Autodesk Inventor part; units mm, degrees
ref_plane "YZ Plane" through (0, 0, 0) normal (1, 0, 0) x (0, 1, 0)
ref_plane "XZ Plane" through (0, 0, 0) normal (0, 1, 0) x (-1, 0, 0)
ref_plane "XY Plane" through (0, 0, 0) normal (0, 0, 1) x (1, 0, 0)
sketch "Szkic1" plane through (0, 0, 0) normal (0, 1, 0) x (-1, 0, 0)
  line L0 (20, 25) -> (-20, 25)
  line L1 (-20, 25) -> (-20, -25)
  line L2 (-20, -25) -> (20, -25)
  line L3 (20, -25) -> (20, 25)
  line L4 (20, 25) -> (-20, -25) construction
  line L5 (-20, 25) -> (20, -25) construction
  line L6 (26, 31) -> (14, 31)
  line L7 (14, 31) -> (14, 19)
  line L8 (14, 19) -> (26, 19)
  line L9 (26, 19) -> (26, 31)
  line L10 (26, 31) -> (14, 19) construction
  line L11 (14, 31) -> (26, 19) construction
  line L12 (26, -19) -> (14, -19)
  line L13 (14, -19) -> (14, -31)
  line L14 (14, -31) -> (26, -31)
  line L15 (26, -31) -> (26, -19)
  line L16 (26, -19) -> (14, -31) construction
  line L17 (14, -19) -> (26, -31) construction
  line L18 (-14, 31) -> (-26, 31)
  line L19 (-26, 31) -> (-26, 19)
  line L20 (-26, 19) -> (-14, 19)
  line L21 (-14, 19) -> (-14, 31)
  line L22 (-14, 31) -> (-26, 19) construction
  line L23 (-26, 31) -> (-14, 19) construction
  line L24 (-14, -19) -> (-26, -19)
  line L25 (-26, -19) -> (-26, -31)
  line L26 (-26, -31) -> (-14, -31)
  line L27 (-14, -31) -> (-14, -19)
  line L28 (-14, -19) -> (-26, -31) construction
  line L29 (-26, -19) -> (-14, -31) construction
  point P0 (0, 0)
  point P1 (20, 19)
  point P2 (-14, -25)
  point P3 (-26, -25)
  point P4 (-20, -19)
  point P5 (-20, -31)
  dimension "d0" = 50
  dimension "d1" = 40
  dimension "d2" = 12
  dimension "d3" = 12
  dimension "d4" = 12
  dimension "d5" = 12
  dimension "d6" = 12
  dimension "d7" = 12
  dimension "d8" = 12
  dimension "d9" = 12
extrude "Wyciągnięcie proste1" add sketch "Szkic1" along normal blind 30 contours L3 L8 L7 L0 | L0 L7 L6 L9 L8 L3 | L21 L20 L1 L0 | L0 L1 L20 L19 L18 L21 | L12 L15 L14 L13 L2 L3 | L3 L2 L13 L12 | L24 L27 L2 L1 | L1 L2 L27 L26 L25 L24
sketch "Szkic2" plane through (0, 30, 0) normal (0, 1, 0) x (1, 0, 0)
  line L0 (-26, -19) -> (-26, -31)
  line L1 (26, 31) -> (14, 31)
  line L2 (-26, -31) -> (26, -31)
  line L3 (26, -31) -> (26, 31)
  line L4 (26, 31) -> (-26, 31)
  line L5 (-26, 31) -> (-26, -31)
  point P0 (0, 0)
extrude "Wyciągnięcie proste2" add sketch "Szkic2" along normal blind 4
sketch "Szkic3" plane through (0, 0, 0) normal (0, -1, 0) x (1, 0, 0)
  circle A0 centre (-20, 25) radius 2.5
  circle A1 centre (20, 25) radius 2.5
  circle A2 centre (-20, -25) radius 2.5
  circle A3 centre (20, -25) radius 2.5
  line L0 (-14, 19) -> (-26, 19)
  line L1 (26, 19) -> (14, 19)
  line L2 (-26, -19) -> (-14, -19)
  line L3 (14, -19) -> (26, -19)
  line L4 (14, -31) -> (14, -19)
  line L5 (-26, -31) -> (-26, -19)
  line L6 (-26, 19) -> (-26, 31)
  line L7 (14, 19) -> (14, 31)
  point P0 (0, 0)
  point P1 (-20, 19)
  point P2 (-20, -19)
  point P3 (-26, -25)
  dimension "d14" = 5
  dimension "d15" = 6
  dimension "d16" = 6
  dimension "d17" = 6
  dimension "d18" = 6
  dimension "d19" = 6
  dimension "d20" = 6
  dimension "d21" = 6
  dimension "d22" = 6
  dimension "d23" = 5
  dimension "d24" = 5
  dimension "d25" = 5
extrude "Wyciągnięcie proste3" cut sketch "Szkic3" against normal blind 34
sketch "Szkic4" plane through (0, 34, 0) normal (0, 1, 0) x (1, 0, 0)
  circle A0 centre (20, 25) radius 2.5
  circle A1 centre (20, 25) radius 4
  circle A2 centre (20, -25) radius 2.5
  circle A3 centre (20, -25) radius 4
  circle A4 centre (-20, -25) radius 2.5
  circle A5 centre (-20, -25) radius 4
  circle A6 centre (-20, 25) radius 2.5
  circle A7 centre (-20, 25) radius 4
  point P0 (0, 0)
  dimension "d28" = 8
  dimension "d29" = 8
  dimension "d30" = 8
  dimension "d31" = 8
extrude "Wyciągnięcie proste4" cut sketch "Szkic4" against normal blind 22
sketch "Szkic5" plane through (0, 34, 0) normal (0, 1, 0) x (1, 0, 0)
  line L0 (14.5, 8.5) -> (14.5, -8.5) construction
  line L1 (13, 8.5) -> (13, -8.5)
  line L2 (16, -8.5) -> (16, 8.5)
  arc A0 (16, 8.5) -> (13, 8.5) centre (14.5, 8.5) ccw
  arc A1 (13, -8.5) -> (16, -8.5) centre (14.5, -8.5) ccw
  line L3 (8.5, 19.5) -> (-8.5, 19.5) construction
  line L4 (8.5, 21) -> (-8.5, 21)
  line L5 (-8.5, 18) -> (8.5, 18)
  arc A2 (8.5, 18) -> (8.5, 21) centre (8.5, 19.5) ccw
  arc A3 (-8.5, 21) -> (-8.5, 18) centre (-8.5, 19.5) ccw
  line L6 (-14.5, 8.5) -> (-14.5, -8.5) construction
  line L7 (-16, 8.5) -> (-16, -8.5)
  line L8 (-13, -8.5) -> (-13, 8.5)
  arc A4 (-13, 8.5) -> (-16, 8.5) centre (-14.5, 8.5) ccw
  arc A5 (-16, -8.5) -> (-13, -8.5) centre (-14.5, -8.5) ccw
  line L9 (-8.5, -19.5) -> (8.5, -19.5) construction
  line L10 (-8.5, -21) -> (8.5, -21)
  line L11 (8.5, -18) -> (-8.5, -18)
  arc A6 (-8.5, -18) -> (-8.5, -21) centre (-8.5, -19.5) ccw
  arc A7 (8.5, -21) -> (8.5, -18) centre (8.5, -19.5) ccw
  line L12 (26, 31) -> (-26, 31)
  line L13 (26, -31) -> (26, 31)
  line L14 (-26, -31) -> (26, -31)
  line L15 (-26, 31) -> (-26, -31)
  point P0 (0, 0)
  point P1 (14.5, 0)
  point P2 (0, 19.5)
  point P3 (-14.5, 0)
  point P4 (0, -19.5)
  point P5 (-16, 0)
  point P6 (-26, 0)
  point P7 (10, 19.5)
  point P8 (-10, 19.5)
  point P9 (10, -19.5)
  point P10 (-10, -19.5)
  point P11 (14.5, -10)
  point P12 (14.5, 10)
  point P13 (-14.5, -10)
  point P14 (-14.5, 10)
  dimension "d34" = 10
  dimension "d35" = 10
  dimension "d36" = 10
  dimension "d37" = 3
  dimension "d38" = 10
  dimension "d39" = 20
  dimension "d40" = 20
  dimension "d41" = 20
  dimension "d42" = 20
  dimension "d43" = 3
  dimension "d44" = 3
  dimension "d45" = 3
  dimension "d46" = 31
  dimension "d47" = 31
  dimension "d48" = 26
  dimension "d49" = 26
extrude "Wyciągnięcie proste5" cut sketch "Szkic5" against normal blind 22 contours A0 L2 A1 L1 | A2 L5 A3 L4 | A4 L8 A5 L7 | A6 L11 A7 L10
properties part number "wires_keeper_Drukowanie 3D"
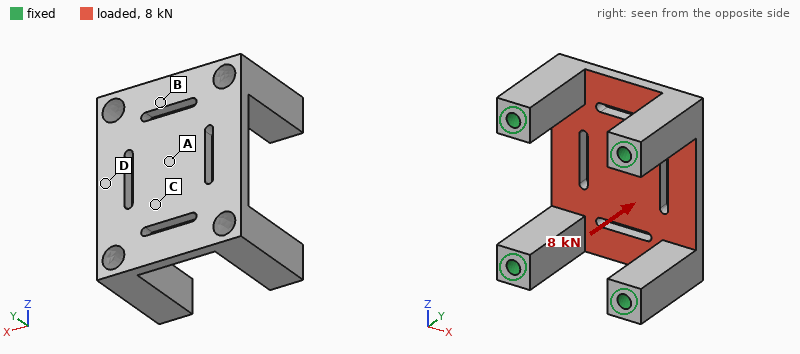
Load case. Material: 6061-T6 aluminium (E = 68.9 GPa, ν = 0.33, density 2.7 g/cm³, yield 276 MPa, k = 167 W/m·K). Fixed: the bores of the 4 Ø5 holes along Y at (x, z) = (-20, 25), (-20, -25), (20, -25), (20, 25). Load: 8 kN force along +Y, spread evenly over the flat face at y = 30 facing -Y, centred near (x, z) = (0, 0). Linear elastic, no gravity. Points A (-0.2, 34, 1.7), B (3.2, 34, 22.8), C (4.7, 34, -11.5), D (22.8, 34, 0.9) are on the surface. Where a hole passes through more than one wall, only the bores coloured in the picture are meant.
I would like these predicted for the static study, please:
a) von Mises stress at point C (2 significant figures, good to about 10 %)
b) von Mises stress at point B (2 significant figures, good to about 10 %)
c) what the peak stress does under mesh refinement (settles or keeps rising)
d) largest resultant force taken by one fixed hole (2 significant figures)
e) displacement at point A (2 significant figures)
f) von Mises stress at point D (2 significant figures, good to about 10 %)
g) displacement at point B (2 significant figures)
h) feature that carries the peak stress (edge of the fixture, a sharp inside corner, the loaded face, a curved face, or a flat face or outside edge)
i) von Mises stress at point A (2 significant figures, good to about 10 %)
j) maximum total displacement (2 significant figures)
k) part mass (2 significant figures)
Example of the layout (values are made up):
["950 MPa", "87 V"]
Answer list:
["81 MPa", "64 MPa", "keeps rising", "2.2 kN", "0.18 mm", "120 MPa", "0.052 mm", "a sharp inside corner", "110 MPa", "0.18 mm", "64 g"]
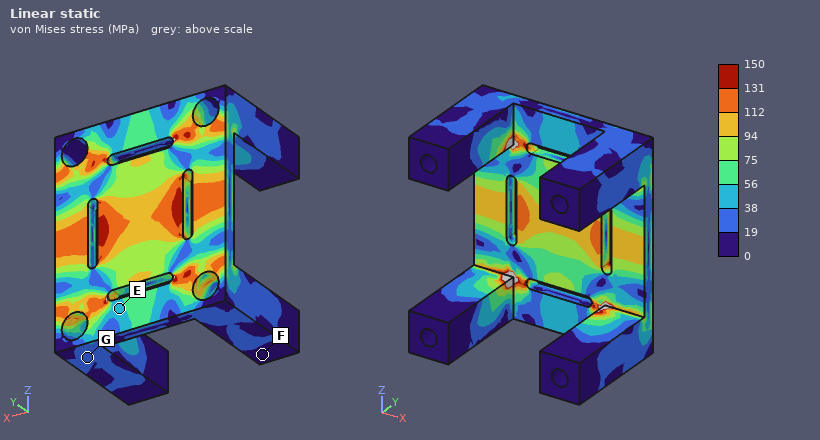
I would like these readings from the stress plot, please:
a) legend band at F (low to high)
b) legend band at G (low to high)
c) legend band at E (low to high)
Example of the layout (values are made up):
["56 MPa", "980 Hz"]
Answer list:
["0 to 19 MPa", "19 to 38 MPa", "38 to 56 MPa"]
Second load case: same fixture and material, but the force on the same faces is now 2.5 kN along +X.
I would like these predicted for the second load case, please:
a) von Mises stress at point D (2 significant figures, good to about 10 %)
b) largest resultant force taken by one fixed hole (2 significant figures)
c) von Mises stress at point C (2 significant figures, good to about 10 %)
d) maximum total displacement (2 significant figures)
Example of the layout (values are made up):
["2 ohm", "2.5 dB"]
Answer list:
["15 MPa", "630 N", "10 MPa", "43 µm"]
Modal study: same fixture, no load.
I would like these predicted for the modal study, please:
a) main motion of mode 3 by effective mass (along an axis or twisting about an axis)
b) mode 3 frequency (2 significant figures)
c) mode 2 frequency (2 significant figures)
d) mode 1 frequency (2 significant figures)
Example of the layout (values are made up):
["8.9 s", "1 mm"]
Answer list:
["along Y", "7800 Hz", "6900 Hz", "6700 Hz"]
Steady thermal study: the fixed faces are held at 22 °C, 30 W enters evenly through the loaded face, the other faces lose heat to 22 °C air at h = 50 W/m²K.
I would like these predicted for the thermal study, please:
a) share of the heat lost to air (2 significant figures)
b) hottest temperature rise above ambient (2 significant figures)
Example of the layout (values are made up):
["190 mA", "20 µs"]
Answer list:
["15 %", "17 K"]
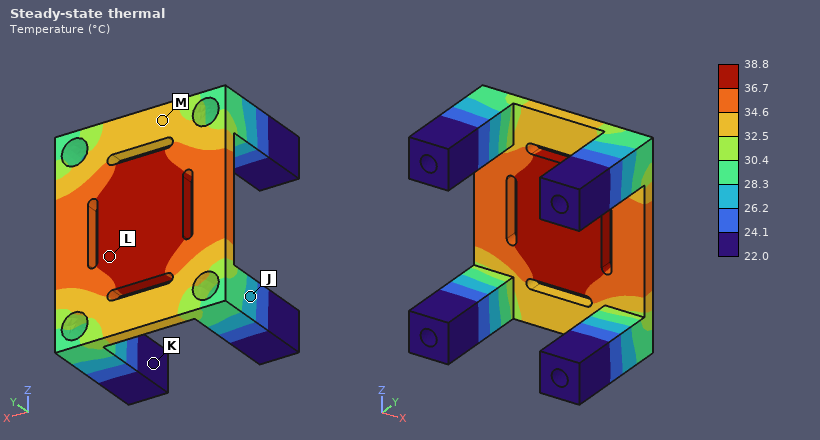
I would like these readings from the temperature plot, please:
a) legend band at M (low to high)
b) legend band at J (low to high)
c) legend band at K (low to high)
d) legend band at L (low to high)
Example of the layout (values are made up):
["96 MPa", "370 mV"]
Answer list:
["32.5 to 34.6 °C", "26.2 to 28.3 °C", "22.0 to 24.1 °C", "36.7 to 38.8 °C"]
